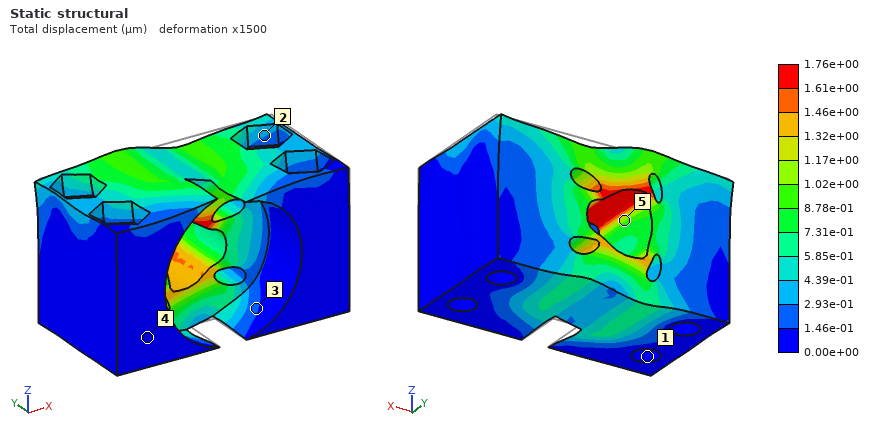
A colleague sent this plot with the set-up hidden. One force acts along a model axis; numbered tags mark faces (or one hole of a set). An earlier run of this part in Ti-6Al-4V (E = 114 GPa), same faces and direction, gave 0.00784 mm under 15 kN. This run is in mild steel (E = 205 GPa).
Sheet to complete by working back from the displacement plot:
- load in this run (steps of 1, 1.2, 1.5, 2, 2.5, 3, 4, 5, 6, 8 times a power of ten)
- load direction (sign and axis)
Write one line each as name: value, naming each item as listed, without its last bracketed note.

load in this run: 6 kN
load direction: -X
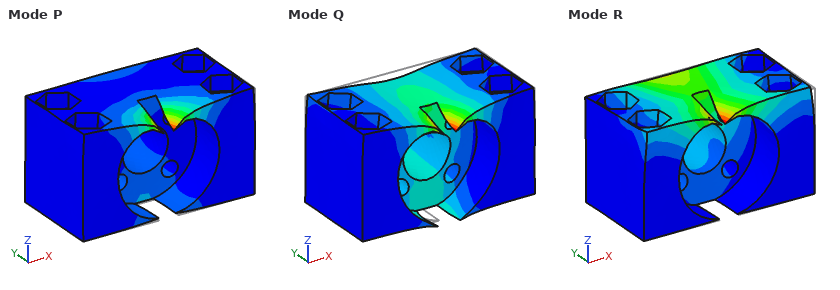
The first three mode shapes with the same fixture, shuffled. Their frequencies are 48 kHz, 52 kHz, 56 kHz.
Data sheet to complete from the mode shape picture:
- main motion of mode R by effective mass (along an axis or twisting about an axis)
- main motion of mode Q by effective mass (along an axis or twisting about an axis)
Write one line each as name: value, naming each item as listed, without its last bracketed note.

main motion of mode R by effective mass: along Y
main motion of mode Q by effective mass: along Z
